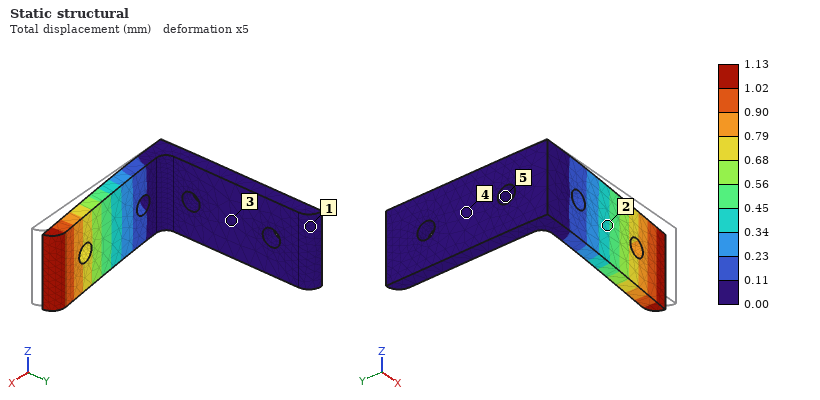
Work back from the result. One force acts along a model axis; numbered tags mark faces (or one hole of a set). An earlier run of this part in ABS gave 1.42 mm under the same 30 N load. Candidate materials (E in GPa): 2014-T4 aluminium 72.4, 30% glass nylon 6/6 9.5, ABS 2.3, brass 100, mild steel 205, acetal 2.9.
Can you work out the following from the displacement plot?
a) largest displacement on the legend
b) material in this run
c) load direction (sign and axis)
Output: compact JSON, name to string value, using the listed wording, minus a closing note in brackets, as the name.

{"largest displacement on the legend": "1.13 mm", "material in this run": "acetal", "load direction": "+Y"}
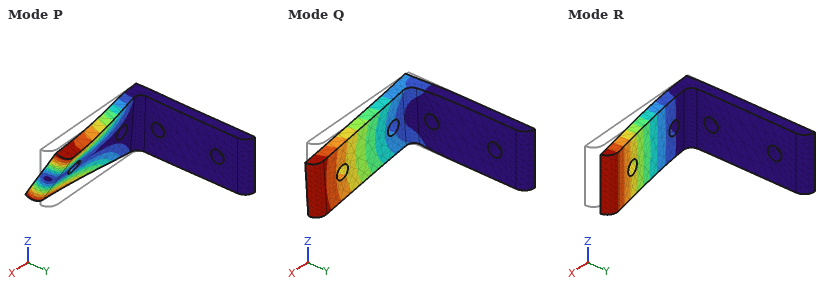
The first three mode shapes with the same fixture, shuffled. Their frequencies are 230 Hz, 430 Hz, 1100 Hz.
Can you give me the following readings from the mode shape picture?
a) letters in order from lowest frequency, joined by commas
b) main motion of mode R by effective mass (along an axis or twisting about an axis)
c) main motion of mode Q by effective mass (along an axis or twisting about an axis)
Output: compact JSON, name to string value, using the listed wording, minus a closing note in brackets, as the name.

{"letters in order from lowest frequency, joined by commas": "R, Q, P", "main motion of mode R by effective mass": "along Y", "main motion of mode Q by effective mass": "along Z"}
